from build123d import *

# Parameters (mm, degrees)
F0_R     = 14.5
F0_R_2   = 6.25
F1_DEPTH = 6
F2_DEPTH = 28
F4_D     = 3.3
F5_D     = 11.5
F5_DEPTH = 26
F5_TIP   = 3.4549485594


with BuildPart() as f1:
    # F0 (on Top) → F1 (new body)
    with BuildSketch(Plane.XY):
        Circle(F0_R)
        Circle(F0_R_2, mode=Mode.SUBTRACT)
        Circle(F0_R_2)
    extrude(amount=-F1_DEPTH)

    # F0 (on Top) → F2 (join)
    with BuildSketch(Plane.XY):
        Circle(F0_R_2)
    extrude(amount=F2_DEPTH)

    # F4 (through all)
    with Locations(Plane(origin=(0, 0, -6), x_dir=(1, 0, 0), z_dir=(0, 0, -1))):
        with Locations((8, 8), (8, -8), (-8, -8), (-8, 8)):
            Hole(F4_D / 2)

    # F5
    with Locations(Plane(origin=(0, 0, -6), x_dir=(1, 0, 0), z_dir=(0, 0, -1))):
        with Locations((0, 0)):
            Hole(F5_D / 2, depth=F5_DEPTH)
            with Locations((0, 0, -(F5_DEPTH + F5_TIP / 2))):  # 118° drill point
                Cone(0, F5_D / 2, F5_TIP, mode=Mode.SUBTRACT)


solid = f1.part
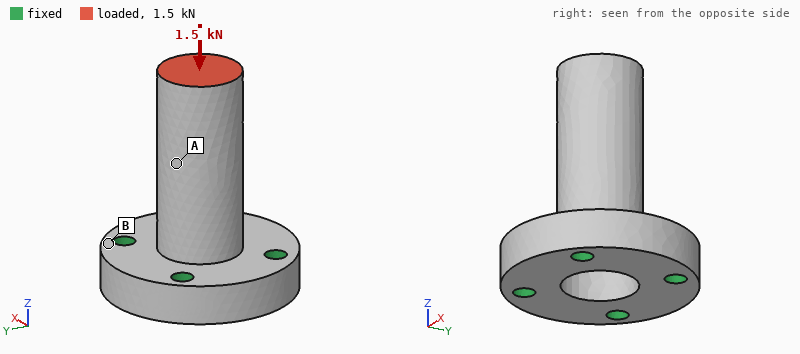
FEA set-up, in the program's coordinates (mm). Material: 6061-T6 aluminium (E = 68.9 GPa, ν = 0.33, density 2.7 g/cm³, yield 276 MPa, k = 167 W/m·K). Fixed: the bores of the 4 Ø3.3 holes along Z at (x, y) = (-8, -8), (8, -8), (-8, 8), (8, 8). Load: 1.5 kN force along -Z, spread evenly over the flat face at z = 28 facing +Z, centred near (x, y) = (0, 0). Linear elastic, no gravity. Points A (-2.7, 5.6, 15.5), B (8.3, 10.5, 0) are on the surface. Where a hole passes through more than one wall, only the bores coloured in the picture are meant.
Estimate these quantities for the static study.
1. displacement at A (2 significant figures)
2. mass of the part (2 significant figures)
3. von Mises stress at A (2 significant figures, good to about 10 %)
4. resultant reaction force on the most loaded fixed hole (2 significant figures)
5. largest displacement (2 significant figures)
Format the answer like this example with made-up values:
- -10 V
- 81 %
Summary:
- 21 µm
- 12 g
- 81 MPa
- 380 N
- 30 µm
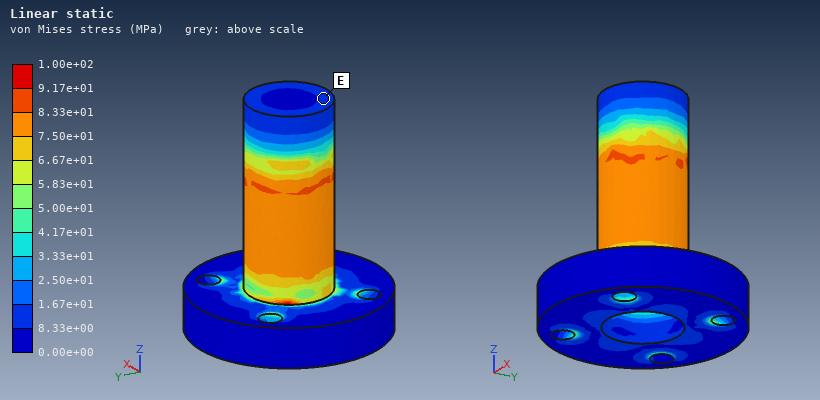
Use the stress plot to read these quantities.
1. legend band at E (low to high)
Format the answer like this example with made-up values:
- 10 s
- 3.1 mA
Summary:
- 8.33e+00 to 1.67e+01 MPa
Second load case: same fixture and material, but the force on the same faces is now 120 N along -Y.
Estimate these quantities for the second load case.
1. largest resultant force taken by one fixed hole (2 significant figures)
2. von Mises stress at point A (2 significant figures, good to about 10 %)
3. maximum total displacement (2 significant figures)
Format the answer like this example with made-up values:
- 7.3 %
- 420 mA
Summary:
- 150 N
- 27 MPa
- 57 µm
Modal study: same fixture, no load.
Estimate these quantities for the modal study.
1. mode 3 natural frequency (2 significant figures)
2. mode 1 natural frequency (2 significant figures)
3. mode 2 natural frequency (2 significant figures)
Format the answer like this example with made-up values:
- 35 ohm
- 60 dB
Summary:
- 18 kHz
- 5300 Hz
- 5300 Hz
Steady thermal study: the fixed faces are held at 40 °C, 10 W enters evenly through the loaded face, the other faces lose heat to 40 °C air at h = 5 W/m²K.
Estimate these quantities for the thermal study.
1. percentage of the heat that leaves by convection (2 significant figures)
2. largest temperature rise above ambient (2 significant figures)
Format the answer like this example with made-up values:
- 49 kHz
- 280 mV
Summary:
- 4.1 %
- 71 K
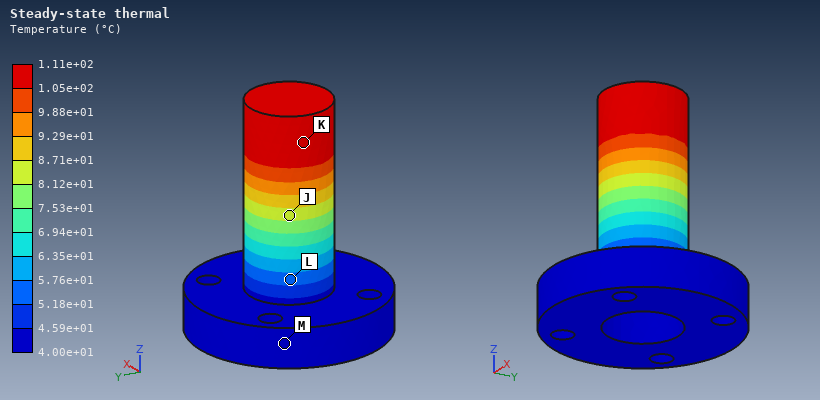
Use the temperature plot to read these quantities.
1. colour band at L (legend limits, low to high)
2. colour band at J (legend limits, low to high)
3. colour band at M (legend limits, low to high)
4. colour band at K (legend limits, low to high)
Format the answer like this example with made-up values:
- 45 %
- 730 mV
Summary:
- 5.18e+01 to 5.76e+01 °C
- 8.12e+01 to 8.71e+01 °C
- 4.00e+01 to 4.59e+01 °C
- 1.05e+02 to 1.11e+02 °C
